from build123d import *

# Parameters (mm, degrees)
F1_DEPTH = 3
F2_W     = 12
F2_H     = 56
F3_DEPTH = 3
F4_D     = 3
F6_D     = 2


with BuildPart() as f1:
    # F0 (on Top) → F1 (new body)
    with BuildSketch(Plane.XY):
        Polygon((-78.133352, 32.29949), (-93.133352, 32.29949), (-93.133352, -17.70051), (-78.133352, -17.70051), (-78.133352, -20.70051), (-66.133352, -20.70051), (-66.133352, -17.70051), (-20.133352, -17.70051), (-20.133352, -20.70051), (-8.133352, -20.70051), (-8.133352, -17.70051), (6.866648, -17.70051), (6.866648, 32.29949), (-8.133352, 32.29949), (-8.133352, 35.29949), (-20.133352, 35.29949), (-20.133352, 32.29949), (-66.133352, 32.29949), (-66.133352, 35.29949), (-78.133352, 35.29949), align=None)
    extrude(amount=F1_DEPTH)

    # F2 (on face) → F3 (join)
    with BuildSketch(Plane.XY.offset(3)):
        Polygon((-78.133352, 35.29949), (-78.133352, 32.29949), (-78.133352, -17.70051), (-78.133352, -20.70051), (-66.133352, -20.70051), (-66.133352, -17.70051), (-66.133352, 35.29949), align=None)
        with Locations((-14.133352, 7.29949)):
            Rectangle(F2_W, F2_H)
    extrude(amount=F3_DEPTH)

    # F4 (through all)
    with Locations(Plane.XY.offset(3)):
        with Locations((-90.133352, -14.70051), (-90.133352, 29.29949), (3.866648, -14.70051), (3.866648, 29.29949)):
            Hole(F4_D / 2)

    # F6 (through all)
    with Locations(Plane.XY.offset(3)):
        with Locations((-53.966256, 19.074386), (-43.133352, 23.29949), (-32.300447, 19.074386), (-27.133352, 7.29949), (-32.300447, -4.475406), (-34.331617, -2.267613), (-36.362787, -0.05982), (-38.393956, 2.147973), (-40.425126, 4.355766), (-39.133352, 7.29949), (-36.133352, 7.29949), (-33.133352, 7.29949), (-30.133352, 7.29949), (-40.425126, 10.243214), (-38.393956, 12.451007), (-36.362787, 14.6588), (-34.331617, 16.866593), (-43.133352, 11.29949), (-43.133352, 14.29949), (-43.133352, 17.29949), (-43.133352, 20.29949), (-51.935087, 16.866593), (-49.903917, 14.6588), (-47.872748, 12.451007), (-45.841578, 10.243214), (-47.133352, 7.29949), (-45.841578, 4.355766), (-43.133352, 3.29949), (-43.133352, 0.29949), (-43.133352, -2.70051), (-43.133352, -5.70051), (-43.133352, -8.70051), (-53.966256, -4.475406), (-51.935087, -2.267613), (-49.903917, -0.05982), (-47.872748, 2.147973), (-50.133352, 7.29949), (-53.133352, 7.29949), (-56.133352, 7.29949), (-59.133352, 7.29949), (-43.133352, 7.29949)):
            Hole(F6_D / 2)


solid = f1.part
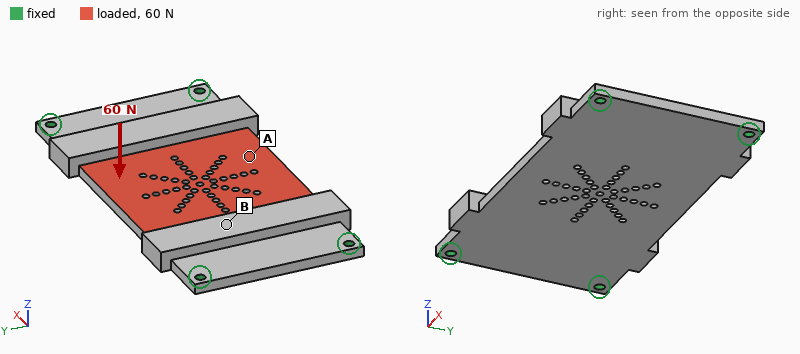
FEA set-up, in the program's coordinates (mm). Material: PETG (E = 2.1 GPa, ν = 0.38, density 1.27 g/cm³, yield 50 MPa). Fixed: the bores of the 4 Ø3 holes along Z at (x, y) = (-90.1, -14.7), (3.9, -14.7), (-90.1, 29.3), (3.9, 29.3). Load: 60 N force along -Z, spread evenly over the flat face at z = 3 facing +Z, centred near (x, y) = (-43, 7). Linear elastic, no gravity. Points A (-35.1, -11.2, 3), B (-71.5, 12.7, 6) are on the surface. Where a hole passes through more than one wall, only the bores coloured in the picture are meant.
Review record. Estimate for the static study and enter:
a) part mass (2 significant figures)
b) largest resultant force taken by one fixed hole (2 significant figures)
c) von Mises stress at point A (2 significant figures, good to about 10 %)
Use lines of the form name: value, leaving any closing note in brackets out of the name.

part mass: 24 g
largest resultant force taken by one fixed hole: 15 N
von Mises stress at point A: 6.1 MPa
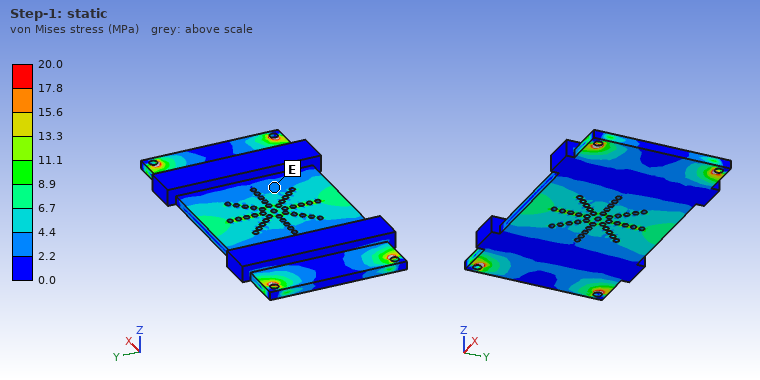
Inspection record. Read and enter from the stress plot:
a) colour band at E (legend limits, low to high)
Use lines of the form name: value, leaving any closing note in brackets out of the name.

colour band at E: 2.2 to 4.4 MPa
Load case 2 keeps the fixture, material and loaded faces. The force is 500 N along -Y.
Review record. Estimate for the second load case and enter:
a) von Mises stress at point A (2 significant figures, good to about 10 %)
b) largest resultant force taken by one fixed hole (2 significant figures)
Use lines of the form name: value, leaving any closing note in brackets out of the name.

von Mises stress at point A: 2.1 MPa
largest resultant force taken by one fixed hole: 170 N
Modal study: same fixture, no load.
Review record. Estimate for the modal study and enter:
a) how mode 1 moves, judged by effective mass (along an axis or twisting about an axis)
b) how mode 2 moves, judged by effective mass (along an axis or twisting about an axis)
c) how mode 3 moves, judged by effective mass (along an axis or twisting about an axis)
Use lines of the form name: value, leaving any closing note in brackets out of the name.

how mode 1 moves, judged by effective mass: along Z
how mode 2 moves, judged by effective mass: twisting about X
how mode 3 moves, judged by effective mass: twisting about Y
